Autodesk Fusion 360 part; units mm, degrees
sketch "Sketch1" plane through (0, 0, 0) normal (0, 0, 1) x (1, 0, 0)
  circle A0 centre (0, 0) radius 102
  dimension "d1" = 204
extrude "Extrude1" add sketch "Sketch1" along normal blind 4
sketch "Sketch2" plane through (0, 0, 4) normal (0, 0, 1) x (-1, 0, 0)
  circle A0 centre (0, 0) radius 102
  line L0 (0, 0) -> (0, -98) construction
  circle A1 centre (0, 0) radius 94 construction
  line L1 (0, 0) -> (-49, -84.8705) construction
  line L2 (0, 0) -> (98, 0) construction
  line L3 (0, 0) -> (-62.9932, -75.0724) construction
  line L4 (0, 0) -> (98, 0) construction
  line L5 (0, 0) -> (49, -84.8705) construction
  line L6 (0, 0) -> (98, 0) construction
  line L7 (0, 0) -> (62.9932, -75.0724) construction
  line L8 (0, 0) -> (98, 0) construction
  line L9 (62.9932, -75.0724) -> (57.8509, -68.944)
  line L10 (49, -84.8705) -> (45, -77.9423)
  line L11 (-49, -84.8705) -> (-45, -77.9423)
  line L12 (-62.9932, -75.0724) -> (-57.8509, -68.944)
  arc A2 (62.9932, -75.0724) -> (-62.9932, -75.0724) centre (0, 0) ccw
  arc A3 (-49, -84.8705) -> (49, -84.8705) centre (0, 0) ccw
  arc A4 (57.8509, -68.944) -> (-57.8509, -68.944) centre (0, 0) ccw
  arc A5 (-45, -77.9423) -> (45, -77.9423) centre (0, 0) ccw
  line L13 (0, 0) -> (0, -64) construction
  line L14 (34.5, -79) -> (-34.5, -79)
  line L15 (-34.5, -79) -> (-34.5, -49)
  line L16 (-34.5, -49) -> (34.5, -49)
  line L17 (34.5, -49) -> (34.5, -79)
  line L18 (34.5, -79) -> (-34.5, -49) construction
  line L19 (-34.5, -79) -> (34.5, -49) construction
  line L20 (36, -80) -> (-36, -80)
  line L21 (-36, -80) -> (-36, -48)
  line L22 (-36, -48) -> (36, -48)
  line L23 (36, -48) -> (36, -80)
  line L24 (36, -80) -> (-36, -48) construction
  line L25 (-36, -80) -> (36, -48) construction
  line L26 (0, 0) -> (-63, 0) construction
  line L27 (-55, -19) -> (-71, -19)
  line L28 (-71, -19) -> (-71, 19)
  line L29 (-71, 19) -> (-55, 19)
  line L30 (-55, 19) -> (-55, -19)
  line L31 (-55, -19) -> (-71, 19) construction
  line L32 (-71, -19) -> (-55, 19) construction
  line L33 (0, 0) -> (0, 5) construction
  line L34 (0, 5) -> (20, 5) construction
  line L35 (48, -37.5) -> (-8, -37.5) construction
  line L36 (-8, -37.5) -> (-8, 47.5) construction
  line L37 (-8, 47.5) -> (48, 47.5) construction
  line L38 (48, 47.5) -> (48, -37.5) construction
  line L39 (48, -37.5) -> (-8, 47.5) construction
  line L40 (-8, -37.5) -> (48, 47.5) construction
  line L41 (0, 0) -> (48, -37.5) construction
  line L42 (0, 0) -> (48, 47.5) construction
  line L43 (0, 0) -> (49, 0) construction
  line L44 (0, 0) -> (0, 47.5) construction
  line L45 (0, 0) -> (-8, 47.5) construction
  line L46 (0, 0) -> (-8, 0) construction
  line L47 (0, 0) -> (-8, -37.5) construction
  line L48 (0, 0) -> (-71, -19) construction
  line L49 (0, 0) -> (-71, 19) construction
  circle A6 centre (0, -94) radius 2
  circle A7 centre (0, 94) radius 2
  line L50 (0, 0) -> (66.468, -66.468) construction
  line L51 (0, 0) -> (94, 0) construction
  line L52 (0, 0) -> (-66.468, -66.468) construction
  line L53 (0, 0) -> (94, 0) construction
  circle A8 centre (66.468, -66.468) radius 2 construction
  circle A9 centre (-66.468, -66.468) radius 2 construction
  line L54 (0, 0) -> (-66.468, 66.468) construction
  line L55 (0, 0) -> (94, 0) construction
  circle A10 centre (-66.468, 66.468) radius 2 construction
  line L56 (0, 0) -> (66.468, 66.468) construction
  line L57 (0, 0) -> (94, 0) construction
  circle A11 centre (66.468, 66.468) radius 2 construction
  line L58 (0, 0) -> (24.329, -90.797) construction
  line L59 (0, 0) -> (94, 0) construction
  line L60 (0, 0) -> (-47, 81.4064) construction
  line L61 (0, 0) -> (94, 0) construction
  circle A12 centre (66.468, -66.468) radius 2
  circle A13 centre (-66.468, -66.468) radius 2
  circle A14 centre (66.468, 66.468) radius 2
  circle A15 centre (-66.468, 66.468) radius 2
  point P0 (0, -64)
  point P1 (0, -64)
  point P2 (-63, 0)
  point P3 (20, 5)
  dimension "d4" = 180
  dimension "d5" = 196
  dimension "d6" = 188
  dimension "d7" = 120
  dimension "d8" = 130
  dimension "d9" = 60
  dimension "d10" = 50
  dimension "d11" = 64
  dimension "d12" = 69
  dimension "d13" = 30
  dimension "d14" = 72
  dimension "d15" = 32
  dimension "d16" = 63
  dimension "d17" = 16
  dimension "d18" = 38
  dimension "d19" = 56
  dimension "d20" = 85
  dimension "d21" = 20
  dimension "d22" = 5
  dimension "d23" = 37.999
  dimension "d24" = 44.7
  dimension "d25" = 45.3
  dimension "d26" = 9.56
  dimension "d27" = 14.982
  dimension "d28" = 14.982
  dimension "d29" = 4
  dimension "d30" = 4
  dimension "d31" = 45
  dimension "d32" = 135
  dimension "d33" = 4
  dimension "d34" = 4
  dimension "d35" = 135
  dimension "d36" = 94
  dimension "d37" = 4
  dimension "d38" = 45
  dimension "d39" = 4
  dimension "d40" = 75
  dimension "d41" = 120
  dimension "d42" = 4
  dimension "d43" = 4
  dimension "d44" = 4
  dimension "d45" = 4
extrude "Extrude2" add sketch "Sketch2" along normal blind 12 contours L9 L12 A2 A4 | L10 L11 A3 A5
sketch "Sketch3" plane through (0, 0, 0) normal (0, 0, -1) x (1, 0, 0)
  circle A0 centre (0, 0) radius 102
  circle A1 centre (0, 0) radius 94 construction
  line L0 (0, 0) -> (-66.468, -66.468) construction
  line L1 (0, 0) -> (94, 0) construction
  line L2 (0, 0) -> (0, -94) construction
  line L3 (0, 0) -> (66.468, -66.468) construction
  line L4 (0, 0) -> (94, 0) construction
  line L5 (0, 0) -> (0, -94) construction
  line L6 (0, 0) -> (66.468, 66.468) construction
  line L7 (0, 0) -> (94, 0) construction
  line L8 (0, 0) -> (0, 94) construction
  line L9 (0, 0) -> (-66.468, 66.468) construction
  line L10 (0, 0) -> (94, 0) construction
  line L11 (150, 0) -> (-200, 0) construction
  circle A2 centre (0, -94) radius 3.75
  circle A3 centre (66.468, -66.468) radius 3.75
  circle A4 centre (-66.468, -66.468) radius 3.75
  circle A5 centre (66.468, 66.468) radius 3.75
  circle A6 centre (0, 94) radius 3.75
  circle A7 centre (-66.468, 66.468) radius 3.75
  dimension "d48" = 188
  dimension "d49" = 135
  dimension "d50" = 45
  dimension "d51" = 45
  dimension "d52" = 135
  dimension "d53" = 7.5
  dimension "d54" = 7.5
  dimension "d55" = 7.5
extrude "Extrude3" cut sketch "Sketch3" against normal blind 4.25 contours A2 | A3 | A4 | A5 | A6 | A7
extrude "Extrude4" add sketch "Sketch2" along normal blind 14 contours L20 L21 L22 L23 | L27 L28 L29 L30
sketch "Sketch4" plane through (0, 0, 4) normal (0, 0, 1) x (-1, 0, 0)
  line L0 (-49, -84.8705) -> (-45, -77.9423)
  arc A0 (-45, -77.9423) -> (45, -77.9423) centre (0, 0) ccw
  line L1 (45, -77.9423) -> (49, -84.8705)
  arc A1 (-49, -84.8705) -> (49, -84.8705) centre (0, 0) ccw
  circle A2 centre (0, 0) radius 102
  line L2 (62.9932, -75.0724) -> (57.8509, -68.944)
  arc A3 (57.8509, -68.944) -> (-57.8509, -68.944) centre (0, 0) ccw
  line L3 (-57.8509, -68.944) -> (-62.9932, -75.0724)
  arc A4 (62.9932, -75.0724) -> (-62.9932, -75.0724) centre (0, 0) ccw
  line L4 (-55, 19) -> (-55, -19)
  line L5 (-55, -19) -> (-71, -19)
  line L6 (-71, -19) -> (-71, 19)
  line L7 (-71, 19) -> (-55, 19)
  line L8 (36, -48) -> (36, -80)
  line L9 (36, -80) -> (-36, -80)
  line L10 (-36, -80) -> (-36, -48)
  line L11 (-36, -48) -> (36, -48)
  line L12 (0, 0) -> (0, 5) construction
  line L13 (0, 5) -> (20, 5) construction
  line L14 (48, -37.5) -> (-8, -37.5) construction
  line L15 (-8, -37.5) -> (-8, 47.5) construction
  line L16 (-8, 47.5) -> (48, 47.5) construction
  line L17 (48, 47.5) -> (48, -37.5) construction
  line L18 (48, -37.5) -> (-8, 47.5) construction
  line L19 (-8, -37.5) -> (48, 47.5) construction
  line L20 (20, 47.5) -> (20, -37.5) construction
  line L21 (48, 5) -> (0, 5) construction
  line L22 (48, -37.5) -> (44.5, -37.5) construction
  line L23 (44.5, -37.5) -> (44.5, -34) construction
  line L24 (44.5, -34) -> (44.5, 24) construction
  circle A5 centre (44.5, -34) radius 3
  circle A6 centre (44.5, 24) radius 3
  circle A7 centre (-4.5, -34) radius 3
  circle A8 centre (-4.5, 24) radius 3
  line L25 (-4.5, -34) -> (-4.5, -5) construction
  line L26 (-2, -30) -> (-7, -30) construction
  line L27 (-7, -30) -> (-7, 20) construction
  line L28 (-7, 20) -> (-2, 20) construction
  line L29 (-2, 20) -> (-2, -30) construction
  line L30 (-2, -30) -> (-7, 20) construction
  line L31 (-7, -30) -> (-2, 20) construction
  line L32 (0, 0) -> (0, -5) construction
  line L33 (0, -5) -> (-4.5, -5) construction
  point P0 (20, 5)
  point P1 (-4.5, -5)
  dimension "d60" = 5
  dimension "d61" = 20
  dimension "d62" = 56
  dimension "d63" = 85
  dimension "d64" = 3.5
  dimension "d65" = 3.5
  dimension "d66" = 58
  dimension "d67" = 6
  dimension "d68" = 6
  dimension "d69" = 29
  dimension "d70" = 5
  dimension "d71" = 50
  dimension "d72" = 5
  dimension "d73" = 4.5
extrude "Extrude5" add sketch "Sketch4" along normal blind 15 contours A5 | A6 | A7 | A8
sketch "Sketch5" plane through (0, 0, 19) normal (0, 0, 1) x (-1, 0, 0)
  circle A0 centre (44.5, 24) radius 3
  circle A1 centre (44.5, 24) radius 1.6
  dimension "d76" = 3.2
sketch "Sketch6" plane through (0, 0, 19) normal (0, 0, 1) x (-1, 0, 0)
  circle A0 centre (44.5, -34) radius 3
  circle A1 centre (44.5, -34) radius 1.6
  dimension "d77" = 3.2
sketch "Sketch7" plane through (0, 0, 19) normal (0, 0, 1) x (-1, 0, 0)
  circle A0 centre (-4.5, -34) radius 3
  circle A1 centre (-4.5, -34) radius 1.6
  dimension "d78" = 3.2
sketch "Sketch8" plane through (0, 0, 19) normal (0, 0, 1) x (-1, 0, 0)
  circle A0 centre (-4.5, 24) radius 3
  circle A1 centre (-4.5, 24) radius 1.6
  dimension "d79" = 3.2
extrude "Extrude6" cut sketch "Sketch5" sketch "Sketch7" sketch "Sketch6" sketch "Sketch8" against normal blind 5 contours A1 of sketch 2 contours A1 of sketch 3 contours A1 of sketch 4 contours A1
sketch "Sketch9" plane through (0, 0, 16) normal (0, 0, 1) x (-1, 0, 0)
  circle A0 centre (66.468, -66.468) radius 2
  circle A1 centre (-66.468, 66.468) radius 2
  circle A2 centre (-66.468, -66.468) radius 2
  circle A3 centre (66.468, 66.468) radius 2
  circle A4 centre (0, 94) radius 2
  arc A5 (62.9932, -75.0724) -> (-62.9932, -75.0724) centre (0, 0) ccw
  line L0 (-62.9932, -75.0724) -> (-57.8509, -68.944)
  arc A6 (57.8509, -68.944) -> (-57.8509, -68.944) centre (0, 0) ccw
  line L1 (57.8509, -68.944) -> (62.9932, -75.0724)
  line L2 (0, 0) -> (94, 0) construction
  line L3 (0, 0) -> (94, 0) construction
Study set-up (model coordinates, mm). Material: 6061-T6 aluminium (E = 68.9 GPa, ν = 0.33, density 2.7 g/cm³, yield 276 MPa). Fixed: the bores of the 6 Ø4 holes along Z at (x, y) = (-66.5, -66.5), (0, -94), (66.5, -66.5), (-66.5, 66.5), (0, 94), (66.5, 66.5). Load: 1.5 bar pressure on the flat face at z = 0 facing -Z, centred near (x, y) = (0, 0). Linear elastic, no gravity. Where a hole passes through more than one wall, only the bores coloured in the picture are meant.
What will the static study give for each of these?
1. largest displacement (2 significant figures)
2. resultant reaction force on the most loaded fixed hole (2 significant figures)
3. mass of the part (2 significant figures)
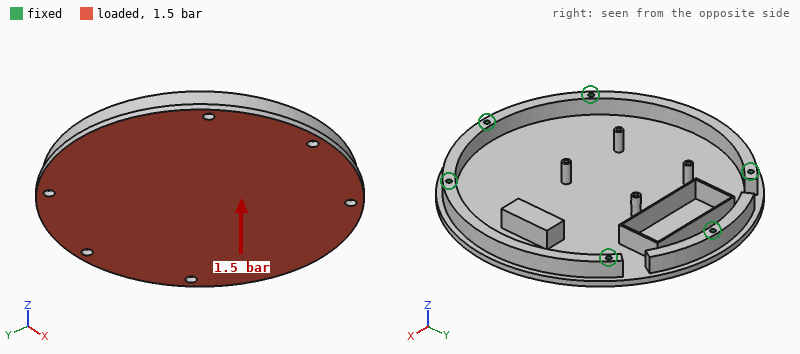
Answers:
0.43 mm
1.3 kN
530 g
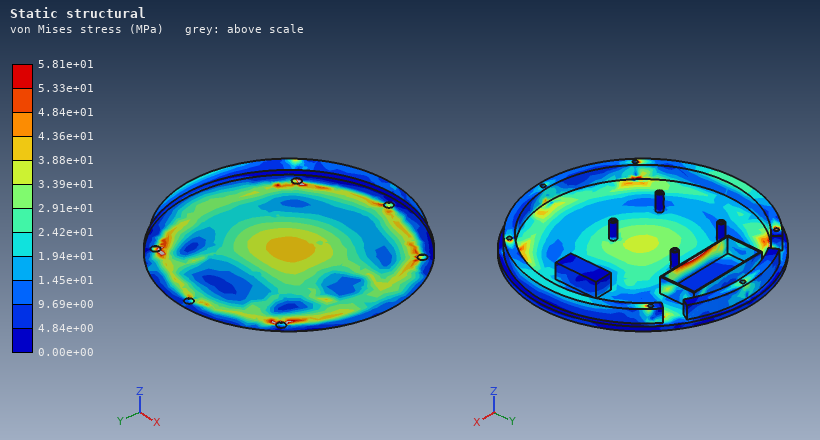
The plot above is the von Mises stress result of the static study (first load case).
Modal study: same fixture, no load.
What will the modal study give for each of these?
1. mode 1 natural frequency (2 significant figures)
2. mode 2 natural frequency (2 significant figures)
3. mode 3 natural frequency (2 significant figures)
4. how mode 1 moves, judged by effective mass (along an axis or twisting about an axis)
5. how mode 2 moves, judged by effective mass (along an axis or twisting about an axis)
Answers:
1100 Hz
2000 Hz
2300 Hz
along Z
twisting about Y
